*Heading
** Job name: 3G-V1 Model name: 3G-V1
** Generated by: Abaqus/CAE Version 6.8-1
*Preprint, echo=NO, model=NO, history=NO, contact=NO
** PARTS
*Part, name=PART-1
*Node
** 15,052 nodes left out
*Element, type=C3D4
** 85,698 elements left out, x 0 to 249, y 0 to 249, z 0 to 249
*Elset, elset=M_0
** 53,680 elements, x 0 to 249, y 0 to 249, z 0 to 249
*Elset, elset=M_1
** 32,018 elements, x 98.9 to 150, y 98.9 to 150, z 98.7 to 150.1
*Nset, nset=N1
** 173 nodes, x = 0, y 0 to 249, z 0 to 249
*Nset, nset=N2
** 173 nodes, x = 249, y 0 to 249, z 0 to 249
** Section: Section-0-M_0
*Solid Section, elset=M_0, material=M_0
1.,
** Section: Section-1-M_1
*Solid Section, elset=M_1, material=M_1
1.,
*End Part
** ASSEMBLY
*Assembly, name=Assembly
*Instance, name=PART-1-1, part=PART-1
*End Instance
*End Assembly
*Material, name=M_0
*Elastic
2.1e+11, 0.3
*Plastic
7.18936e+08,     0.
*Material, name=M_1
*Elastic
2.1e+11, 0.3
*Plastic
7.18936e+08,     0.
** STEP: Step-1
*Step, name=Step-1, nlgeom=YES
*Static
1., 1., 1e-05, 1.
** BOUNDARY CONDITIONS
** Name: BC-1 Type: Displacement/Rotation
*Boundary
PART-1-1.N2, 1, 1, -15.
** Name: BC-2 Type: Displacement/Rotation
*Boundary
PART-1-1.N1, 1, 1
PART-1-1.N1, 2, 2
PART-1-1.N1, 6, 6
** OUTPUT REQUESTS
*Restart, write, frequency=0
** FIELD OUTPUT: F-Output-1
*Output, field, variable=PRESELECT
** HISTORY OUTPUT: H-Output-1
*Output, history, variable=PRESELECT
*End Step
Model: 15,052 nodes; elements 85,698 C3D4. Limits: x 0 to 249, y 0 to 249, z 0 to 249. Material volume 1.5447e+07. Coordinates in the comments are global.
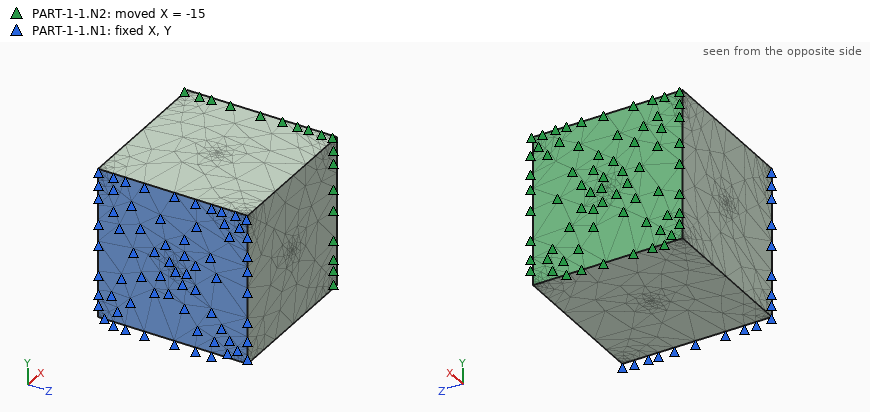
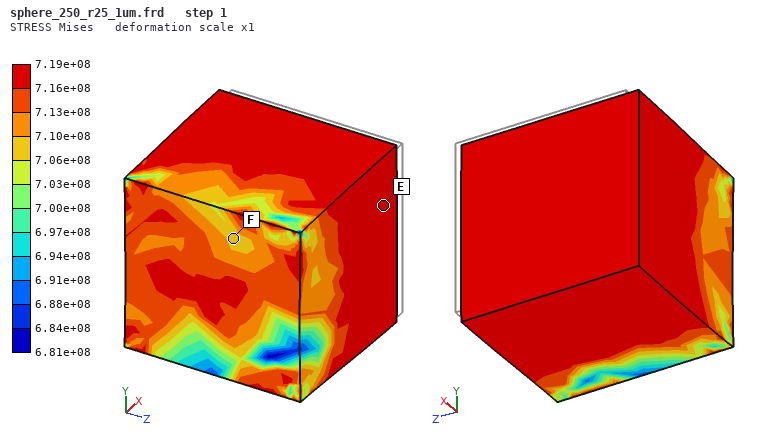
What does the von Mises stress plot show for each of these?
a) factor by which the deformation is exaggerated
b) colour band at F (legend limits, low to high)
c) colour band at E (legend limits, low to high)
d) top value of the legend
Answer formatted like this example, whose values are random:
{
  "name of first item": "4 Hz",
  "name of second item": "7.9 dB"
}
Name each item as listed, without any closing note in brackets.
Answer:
{
  "factor by which the deformation is exaggerated": "1",
  "colour band at F": "7.06e+08 to 7.10e+08",
  "colour band at E": "7.16e+08 to 7.19e+08",
  "top value of the legend": "7.19e+08"
}
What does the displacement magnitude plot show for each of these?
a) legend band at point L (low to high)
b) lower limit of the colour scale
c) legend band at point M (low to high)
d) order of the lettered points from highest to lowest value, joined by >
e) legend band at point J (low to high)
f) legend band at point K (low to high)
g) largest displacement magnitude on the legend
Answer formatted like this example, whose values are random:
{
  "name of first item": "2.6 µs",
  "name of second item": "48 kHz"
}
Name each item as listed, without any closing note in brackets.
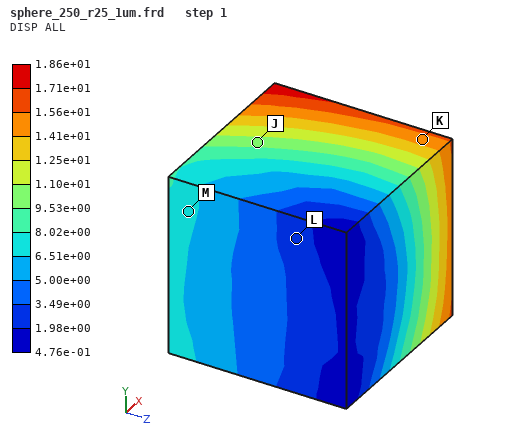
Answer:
{
  "legend band at point L": "1.98e+00 to 3.49e+00",
  "lower limit of the colour scale": "4.76e-01",
  "legend band at point M": "6.51e+00 to 8.02e+00",
  "order of the lettered points from highest to lowest value, joined by >": "K > J > M > L",
  "legend band at point J": "9.53e+00 to 1.10e+01",
  "legend band at point K": "1.41e+01 to 1.56e+01",
  "largest displacement magnitude on the legend": "1.86e+01"
}
